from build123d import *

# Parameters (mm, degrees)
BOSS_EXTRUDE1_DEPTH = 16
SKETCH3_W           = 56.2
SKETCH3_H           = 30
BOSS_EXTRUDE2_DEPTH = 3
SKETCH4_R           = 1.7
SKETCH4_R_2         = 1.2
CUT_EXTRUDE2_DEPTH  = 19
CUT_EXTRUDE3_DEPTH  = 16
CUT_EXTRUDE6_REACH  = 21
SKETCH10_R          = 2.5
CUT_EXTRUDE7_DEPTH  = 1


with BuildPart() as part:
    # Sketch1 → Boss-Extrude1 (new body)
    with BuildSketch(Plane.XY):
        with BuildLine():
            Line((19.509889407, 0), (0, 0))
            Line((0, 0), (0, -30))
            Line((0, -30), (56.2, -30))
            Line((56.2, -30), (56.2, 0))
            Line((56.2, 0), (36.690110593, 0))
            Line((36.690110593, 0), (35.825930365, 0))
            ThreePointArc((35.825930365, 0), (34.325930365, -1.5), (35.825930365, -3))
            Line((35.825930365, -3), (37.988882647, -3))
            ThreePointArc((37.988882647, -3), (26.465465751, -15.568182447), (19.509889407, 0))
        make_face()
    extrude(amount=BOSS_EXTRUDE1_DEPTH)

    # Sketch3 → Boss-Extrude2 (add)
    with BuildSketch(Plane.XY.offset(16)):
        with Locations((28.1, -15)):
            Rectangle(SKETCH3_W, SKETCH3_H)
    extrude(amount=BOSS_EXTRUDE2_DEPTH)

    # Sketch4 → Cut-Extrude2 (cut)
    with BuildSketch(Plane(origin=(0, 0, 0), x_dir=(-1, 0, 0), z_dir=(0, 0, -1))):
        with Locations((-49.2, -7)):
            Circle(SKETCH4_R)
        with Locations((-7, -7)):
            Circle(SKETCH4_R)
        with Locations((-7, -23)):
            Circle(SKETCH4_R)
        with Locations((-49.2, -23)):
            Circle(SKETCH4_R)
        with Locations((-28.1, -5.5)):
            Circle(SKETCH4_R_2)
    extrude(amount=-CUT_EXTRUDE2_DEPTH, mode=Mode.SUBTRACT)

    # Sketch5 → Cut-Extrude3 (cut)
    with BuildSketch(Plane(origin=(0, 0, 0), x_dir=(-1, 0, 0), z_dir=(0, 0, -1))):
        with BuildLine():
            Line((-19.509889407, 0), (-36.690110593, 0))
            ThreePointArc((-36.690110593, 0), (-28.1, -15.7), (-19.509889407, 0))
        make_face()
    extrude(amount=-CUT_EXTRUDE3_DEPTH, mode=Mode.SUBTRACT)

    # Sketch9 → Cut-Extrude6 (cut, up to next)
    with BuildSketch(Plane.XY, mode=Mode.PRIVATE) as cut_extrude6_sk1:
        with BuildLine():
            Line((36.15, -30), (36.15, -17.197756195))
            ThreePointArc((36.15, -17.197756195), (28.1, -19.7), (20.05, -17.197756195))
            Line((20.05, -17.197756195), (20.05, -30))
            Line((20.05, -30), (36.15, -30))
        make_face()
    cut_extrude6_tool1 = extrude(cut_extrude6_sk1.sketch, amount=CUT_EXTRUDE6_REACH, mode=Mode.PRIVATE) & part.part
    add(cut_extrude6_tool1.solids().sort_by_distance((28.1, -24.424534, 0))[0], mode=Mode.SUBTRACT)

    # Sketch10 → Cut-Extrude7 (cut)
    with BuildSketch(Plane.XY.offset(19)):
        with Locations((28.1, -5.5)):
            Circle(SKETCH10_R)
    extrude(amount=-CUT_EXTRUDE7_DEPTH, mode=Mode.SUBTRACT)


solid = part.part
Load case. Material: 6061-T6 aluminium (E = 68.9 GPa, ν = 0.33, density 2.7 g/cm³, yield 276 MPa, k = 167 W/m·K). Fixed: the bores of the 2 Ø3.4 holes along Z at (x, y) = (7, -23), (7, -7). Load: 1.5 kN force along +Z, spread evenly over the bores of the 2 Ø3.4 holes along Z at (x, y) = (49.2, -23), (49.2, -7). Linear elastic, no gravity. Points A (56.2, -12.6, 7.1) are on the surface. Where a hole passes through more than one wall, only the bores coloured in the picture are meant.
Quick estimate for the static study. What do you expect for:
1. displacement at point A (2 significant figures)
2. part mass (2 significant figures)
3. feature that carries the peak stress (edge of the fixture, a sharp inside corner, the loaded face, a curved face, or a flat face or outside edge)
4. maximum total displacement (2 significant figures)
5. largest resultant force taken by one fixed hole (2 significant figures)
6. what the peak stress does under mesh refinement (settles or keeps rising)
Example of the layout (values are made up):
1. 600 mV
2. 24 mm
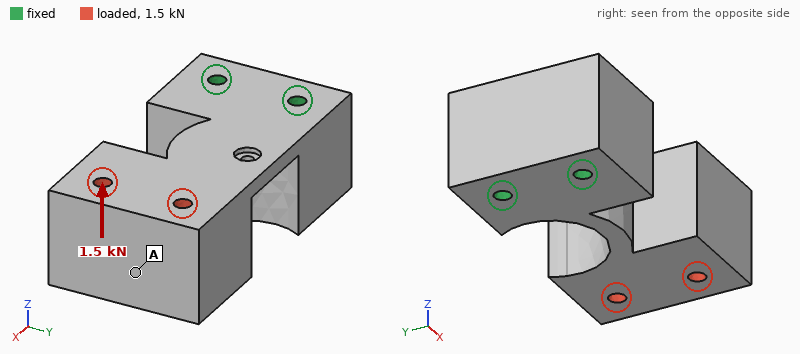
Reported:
1. 0.22 mm
2. 64 g
3. a sharp inside corner
4. 0.26 mm
5. 780 N
6. keeps rising
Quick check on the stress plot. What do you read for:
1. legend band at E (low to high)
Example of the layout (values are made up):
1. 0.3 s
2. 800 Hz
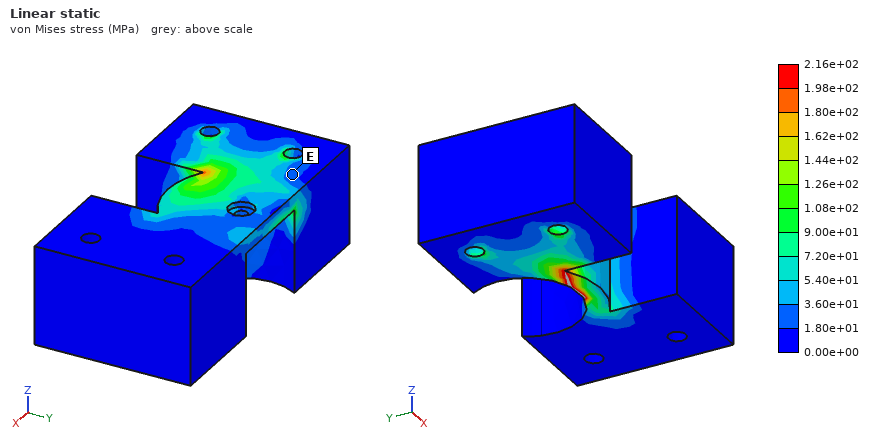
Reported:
1. 1.80e+01 to 3.60e+01 MPa
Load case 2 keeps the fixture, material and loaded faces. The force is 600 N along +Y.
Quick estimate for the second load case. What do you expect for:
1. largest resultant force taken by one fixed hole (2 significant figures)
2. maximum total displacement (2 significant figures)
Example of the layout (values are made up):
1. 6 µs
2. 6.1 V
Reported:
1. 1.5 kN
2. 0.13 mm
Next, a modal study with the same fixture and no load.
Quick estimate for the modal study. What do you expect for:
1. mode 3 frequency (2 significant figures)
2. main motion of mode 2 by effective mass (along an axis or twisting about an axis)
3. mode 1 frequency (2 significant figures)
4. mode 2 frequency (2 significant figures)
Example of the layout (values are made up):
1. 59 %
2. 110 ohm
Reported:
1. 4800 Hz
2. along Z
3. 2400 Hz
4. 3100 Hz
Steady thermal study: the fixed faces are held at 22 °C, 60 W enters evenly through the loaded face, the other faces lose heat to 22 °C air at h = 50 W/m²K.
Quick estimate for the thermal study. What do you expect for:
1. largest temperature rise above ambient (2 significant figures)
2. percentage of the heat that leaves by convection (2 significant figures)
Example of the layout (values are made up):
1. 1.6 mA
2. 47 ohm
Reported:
1. 69 K
2. 20 %
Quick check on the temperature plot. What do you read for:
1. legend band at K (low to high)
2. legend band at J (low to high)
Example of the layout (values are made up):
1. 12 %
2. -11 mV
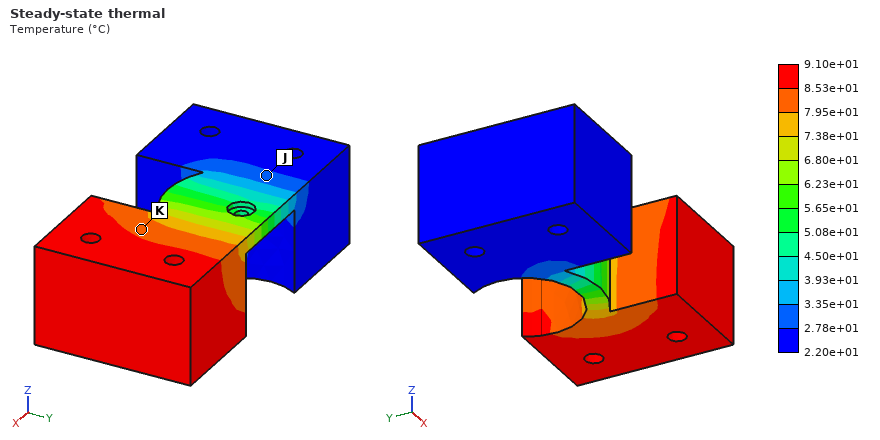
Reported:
1. 7.95e+01 to 8.53e+01 °C
2. 2.78e+01 to 3.35e+01 °C
